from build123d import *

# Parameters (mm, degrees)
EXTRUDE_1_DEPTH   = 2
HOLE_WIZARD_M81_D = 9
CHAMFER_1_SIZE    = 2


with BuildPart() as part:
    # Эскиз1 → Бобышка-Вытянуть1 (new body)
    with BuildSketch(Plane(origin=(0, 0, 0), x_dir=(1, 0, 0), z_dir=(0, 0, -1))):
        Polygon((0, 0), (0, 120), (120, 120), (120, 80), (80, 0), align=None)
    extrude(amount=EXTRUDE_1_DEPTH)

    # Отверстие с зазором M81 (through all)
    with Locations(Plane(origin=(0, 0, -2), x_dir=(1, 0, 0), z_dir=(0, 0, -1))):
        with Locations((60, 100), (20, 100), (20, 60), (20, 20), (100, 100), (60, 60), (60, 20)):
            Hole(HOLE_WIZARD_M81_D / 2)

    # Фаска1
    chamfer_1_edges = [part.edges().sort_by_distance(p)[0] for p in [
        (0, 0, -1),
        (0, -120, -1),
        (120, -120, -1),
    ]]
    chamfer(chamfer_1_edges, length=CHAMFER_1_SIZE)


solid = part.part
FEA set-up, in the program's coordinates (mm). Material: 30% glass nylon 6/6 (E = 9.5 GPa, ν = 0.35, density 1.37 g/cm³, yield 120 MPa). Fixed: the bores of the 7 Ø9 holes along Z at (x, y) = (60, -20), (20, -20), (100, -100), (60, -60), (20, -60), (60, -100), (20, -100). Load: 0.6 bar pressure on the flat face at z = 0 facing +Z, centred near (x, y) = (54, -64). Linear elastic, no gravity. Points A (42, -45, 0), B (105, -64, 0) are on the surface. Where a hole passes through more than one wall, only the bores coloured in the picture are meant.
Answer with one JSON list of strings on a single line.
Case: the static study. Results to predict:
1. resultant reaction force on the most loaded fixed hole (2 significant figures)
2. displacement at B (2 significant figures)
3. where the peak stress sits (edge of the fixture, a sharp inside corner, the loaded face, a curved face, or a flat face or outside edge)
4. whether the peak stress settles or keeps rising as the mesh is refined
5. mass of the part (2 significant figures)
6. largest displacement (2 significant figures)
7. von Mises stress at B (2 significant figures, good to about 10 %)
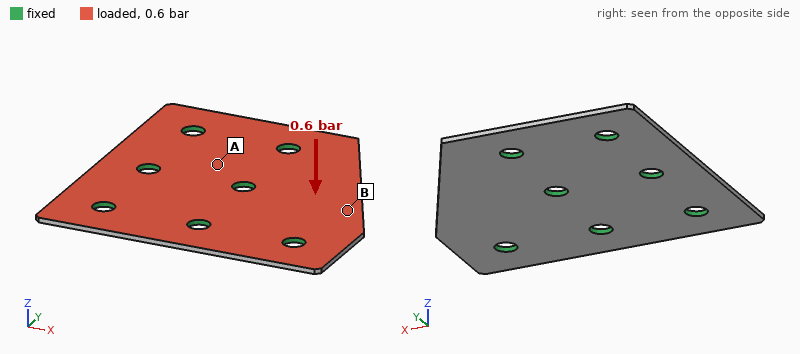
["130 N", "1.1 mm", "edge of the fixture", "keeps rising", "34 g", "1.6 mm", "14 MPa"]
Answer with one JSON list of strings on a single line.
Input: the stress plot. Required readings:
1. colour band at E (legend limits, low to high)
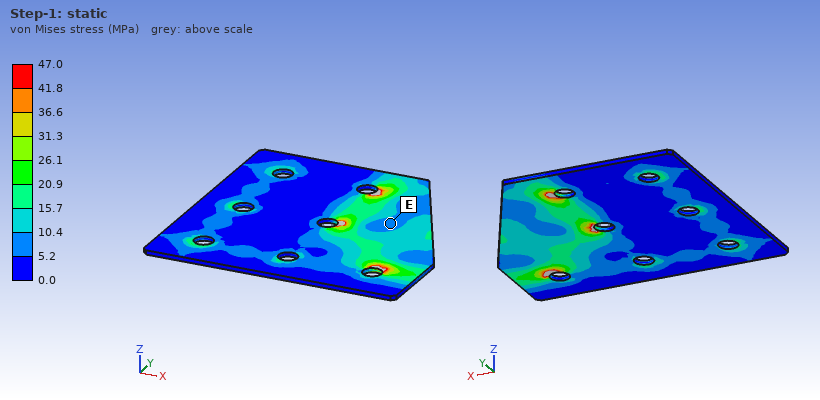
["5.2 to 10.4 MPa"]
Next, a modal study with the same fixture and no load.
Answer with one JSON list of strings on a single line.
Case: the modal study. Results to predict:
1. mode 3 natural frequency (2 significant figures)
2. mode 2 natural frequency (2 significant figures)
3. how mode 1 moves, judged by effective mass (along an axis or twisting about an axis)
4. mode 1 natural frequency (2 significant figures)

["2100 Hz", "1500 Hz", "along Z", "810 Hz"]
